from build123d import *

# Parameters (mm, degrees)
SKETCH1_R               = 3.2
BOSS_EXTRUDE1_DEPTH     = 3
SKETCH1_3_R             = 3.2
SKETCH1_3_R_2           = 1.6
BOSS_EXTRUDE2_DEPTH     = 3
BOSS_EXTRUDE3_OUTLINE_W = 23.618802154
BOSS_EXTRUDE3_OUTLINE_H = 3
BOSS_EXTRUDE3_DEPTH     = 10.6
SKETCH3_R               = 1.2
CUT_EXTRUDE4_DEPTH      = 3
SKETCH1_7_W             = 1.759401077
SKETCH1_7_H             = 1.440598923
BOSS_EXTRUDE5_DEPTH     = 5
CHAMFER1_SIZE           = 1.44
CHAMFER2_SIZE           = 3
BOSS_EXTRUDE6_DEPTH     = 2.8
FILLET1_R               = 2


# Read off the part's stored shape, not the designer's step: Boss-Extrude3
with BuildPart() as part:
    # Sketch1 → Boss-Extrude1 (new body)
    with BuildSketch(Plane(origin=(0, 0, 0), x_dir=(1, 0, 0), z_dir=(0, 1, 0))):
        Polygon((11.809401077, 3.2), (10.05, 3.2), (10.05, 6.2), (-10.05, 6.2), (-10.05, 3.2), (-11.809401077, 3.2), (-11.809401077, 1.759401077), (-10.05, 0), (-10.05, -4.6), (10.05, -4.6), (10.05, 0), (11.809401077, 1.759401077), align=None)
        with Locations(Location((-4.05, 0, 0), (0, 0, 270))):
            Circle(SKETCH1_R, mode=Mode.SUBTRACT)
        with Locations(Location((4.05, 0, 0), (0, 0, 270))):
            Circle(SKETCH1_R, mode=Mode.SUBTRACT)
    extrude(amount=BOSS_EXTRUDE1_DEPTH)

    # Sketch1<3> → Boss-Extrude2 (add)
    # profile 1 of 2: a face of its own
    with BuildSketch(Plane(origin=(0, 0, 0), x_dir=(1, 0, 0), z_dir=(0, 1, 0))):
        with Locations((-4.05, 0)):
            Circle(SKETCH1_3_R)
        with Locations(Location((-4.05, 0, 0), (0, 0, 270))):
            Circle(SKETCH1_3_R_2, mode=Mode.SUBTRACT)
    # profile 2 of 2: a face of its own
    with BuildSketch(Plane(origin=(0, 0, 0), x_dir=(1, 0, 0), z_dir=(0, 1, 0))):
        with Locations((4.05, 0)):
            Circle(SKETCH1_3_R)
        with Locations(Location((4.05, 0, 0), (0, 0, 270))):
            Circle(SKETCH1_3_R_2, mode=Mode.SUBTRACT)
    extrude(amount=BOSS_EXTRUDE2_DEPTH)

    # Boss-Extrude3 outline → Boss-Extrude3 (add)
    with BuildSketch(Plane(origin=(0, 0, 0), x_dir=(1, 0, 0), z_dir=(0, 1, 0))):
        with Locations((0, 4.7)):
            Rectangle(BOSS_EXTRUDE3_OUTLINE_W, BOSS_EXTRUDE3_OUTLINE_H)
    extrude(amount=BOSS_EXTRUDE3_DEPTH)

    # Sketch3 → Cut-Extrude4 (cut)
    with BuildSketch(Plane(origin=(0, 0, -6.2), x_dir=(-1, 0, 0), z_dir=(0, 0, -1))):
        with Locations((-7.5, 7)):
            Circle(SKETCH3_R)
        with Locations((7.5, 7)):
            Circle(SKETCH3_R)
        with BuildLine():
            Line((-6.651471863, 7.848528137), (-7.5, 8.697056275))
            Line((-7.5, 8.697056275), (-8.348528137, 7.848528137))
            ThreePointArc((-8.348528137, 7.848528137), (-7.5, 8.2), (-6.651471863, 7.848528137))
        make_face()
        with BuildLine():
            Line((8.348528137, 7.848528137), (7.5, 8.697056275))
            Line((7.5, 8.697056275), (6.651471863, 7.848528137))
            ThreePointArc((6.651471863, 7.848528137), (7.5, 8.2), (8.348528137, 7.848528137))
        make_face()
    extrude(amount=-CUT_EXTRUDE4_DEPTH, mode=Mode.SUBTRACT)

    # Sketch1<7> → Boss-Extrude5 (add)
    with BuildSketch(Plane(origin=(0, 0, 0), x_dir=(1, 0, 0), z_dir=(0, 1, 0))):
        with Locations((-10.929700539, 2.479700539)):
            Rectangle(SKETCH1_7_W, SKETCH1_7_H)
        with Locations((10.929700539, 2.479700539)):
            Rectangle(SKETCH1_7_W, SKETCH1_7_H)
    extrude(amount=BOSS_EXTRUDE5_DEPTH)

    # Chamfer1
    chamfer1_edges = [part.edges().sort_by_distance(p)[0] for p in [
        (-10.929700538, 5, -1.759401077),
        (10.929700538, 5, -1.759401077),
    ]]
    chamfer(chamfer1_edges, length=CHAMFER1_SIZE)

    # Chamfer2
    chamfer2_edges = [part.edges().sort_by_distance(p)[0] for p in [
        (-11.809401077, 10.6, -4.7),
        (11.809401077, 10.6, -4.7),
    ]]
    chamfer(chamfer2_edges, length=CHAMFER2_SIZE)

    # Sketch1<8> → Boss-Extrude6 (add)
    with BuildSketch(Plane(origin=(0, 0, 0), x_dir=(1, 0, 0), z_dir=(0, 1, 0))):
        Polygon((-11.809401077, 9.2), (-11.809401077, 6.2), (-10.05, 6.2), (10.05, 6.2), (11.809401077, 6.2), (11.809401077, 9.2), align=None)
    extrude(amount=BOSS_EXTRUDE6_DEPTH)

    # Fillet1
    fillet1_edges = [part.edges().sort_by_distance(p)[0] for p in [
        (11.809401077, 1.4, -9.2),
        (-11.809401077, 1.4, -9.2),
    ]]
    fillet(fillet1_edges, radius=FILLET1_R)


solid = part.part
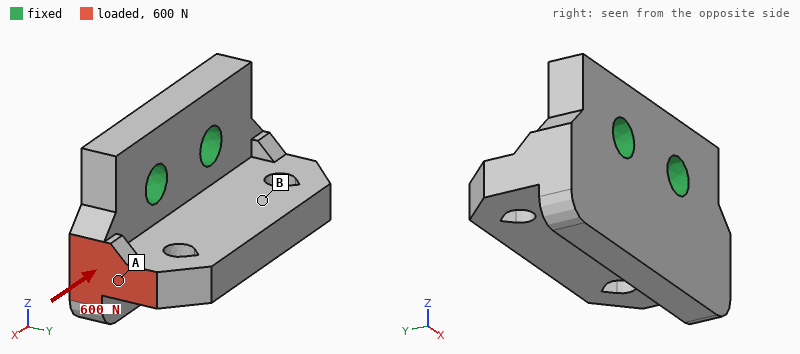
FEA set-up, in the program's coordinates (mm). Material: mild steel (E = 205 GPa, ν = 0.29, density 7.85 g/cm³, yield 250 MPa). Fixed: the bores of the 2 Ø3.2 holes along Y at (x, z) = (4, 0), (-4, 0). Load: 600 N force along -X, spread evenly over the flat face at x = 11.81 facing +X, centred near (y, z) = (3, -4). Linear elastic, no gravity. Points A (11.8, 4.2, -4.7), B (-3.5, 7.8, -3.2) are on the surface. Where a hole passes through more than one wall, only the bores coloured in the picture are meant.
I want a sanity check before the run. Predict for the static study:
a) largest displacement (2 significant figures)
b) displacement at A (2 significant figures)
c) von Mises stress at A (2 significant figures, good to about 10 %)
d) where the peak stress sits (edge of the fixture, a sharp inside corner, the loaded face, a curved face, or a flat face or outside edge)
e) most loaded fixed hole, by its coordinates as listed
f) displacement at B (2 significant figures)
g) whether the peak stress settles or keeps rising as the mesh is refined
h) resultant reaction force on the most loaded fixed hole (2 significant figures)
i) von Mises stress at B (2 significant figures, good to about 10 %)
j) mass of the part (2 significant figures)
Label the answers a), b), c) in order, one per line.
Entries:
a) 2.4 µm
b) 2.1 µm
c) 16 MPa
d) edge of the fixture
e) (4, 0)
f) 1.2 µm
g) keeps rising
h) 440 N
i) 5.4 MPa
j) 11 g
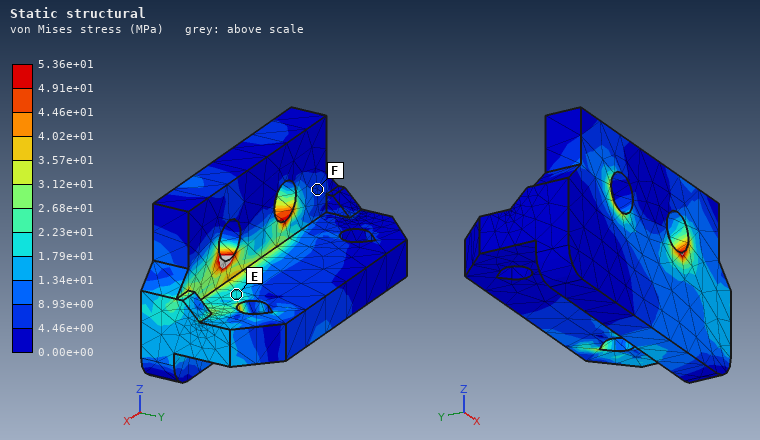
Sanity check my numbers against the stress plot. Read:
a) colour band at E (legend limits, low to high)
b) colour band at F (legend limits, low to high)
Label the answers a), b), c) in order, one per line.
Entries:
a) 1.79e+01 to 2.23e+01 MPa
b) 4.46e+00 to 8.93e+00 MPa
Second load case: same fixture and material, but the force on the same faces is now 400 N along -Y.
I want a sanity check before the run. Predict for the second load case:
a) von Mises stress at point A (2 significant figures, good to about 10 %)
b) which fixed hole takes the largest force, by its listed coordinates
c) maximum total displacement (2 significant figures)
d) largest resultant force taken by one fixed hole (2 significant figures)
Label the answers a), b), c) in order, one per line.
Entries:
a) 31 MPa
b) (4, 0)
c) 10 µm
d) 580 N
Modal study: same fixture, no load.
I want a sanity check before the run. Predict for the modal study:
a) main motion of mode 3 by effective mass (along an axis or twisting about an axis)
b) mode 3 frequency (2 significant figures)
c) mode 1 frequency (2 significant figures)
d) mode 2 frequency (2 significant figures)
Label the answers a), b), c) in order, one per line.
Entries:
a) along X
b) 35 kHz
c) 17 kHz
d) 23 kHz
